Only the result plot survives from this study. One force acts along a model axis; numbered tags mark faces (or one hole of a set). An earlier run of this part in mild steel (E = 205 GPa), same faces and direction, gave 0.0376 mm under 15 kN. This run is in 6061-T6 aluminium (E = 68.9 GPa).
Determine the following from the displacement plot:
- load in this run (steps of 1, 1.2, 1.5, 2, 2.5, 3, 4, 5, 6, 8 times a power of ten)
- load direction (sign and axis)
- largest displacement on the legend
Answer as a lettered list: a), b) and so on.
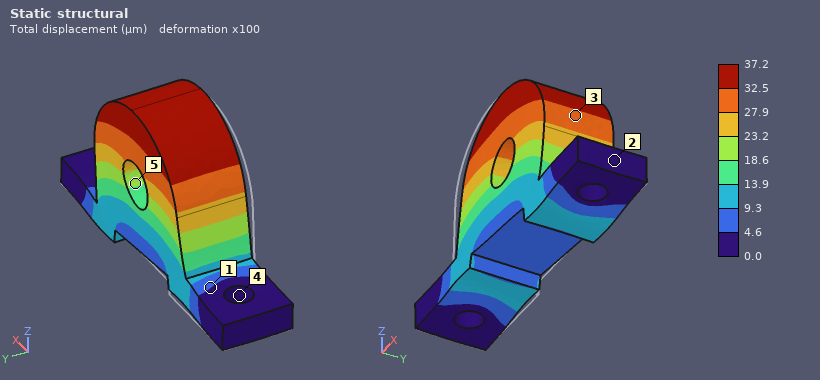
a) 5 kN
b) +X
c) 37.2 µm
